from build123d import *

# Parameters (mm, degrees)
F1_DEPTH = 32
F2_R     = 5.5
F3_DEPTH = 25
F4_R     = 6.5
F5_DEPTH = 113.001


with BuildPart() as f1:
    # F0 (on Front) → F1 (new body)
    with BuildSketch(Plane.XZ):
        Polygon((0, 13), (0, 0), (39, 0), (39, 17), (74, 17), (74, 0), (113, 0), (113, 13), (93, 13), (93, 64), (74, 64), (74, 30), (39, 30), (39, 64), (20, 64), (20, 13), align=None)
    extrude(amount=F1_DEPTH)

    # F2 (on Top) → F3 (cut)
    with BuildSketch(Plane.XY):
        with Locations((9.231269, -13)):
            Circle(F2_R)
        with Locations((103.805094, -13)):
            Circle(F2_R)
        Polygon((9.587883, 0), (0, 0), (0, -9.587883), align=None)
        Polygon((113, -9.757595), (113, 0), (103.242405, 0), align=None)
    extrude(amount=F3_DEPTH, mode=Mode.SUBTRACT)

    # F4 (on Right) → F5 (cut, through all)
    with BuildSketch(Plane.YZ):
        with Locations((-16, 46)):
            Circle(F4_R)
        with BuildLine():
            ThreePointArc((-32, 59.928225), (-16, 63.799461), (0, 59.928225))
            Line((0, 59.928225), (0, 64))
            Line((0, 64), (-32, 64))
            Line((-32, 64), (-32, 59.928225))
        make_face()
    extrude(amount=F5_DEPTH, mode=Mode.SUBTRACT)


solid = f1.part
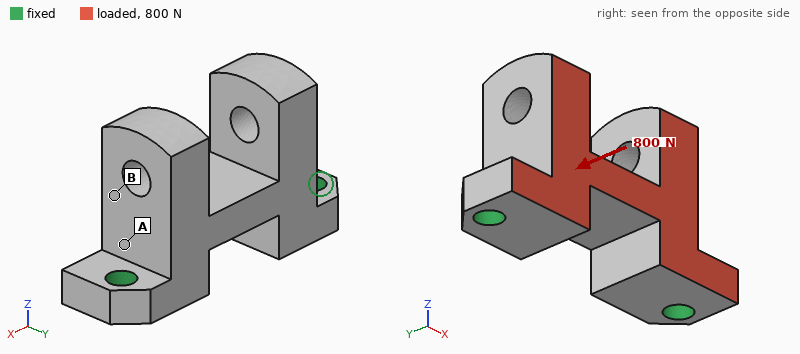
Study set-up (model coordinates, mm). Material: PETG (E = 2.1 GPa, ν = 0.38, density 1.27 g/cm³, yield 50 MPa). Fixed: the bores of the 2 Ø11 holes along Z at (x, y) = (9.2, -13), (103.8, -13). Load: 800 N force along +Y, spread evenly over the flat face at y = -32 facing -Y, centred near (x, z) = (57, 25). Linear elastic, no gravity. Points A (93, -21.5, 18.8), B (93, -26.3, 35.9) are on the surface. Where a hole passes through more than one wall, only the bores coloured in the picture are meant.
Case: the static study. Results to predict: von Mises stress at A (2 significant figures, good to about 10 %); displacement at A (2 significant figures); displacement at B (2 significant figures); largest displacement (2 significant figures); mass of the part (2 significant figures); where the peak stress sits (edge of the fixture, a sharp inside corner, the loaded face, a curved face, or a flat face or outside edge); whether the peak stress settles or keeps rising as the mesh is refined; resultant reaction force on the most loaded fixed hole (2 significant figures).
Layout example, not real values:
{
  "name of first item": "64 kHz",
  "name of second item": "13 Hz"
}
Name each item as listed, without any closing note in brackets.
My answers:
{
  "von Mises stress at A": "2.6 MPa",
  "displacement at A": "0.11 mm",
  "displacement at B": "0.25 mm",
  "largest displacement": "0.44 mm",
  "mass of the part": "130 g",
  "where the peak stress sits": "edge of the fixture",
  "whether the peak stress settles or keeps rising as the mesh is refined": "keeps rising",
  "resultant reaction force on the most loaded fixed hole": "400 N"
}
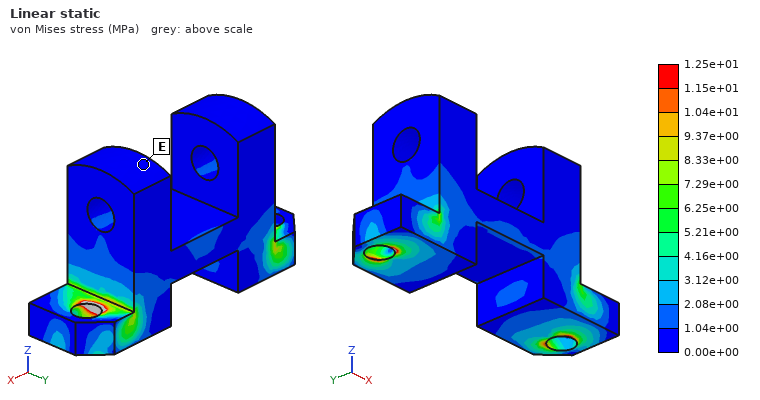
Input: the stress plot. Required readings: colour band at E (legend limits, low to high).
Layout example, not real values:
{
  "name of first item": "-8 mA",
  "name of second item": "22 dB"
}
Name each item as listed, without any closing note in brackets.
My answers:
{
  "colour band at E": "0.00e+00 to 1.04e+00 MPa"
}
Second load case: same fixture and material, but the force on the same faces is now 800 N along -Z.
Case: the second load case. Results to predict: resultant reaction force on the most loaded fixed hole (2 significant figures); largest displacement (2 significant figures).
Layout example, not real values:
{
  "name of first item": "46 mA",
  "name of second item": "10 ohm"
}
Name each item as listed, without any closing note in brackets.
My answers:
{
  "resultant reaction force on the most loaded fixed hole": "460 N",
  "largest displacement": "0.35 mm"
}
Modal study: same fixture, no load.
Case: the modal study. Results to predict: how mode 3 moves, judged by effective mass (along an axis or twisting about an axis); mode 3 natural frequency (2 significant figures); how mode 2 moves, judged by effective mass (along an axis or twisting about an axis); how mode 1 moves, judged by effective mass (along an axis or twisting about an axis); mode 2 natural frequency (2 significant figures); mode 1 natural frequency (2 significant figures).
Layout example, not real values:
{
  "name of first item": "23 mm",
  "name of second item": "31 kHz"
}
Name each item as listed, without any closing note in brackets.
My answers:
{
  "how mode 3 moves, judged by effective mass": "along X",
  "mode 3 natural frequency": "1400 Hz",
  "how mode 2 moves, judged by effective mass": "twisting about Z",
  "how mode 1 moves, judged by effective mass": "along Y",
  "mode 2 natural frequency": "1100 Hz",
  "mode 1 natural frequency": "730 Hz"
}
